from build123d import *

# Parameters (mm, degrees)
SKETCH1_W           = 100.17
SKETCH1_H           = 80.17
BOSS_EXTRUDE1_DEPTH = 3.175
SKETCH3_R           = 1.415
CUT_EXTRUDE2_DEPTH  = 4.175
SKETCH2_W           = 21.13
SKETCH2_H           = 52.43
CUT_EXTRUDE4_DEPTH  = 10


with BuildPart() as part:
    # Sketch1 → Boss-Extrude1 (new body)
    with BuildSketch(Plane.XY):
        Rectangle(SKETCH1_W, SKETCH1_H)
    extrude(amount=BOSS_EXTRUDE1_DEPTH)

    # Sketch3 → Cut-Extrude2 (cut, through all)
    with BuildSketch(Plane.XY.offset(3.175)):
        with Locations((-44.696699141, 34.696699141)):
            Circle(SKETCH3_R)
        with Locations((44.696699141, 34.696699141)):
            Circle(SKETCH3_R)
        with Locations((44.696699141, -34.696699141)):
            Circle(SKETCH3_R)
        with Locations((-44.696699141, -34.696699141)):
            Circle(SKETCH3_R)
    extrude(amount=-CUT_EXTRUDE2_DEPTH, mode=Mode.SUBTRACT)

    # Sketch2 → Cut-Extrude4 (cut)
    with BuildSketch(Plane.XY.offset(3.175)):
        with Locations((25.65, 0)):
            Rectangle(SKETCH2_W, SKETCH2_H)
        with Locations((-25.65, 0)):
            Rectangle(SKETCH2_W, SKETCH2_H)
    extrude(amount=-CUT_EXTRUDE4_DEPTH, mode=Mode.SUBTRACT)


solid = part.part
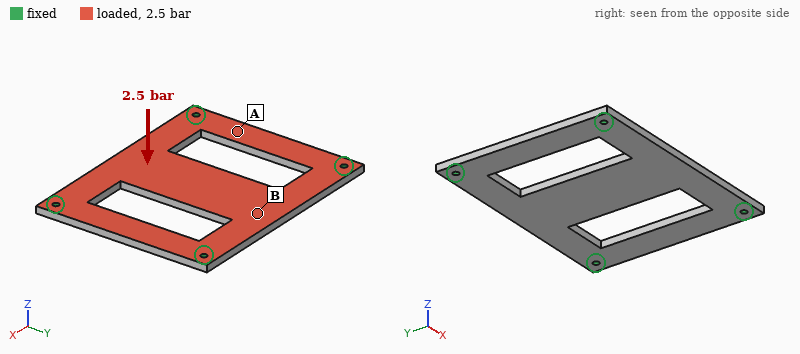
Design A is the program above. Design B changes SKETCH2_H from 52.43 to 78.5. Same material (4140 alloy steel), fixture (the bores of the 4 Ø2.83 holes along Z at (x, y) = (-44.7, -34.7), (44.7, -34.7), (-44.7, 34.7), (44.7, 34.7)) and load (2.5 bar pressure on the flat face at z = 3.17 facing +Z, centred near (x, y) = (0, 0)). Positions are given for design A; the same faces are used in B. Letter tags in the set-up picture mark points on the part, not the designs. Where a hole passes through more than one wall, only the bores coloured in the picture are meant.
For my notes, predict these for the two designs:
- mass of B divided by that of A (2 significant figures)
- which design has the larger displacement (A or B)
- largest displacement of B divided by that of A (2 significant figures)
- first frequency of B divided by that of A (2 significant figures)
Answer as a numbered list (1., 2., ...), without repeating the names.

1. 0.81
2. B
3. 4.1
4. 0.19
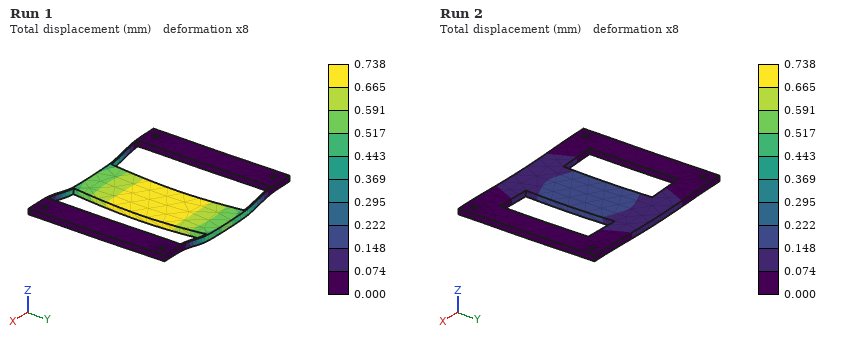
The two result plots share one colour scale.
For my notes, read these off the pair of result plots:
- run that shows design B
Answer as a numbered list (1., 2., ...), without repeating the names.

1. Run 1
